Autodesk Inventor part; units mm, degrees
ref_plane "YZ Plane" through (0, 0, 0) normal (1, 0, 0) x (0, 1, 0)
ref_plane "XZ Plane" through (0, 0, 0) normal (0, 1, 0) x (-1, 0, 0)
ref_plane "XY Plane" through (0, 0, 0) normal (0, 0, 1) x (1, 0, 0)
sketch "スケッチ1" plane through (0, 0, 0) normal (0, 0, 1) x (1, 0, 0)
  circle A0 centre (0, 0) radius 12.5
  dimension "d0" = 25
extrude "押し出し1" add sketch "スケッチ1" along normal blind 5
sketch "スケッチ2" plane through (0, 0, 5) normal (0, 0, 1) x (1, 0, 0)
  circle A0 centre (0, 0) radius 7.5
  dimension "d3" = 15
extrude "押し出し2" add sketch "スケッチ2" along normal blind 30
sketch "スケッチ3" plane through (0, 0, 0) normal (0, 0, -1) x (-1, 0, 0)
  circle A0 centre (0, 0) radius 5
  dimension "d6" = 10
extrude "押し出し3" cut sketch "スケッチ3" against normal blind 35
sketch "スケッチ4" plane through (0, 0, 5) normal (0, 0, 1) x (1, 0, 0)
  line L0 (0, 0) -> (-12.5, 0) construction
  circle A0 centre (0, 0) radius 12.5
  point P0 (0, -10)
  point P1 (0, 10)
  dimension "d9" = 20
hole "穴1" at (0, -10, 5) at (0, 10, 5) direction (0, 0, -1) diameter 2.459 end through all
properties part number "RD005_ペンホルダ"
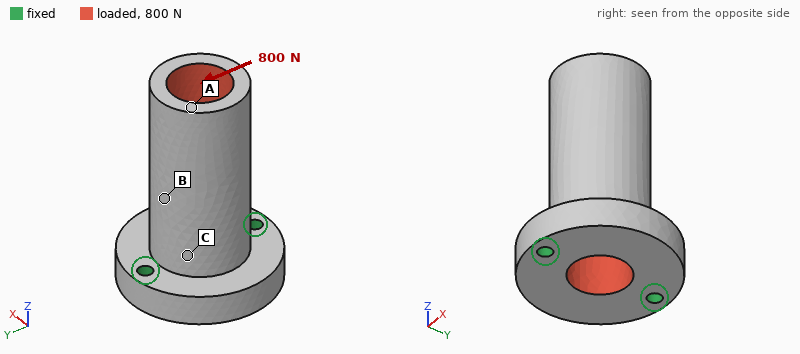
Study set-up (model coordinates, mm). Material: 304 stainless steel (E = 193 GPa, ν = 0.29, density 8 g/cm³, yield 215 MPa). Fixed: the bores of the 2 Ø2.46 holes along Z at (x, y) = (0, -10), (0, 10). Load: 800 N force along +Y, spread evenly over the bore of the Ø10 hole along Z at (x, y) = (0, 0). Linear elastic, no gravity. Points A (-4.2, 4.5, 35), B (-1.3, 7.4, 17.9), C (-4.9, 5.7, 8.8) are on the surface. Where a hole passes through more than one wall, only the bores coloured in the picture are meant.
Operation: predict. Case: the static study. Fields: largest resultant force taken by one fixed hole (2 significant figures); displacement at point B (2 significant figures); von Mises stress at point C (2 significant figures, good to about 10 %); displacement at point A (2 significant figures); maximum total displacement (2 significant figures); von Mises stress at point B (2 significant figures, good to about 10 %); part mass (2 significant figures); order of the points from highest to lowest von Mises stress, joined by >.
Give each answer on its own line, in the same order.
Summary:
800 N
6.5 µm
22 MPa
14 µm
14 µm
12 MPa
40 g
C > B > A
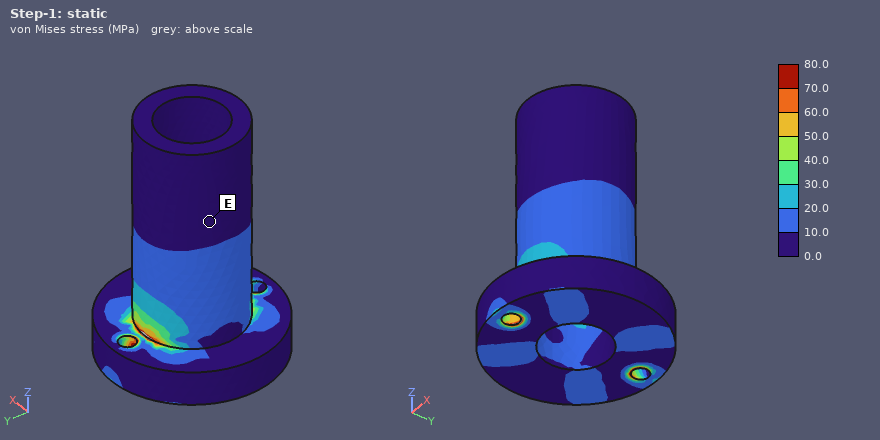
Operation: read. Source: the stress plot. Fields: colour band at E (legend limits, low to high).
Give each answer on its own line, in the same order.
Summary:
0.0 to 10.0 MPa
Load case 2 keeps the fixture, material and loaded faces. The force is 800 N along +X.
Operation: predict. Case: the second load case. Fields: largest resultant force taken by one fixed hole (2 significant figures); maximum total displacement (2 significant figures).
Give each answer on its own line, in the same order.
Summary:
400 N
43 µm
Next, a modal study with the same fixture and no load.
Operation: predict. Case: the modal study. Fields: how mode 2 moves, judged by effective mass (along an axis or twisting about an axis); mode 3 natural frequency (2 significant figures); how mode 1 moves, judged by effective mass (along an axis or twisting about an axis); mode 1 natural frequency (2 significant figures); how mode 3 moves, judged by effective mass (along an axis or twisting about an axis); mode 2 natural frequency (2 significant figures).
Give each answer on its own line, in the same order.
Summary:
along Y
21 kHz
along X
4900 Hz
along Z
8700 Hz
